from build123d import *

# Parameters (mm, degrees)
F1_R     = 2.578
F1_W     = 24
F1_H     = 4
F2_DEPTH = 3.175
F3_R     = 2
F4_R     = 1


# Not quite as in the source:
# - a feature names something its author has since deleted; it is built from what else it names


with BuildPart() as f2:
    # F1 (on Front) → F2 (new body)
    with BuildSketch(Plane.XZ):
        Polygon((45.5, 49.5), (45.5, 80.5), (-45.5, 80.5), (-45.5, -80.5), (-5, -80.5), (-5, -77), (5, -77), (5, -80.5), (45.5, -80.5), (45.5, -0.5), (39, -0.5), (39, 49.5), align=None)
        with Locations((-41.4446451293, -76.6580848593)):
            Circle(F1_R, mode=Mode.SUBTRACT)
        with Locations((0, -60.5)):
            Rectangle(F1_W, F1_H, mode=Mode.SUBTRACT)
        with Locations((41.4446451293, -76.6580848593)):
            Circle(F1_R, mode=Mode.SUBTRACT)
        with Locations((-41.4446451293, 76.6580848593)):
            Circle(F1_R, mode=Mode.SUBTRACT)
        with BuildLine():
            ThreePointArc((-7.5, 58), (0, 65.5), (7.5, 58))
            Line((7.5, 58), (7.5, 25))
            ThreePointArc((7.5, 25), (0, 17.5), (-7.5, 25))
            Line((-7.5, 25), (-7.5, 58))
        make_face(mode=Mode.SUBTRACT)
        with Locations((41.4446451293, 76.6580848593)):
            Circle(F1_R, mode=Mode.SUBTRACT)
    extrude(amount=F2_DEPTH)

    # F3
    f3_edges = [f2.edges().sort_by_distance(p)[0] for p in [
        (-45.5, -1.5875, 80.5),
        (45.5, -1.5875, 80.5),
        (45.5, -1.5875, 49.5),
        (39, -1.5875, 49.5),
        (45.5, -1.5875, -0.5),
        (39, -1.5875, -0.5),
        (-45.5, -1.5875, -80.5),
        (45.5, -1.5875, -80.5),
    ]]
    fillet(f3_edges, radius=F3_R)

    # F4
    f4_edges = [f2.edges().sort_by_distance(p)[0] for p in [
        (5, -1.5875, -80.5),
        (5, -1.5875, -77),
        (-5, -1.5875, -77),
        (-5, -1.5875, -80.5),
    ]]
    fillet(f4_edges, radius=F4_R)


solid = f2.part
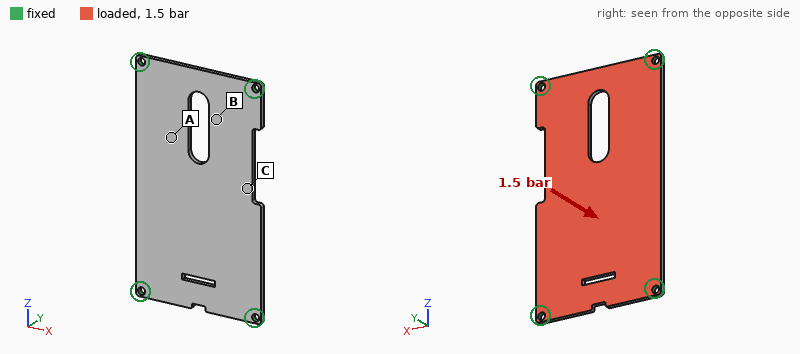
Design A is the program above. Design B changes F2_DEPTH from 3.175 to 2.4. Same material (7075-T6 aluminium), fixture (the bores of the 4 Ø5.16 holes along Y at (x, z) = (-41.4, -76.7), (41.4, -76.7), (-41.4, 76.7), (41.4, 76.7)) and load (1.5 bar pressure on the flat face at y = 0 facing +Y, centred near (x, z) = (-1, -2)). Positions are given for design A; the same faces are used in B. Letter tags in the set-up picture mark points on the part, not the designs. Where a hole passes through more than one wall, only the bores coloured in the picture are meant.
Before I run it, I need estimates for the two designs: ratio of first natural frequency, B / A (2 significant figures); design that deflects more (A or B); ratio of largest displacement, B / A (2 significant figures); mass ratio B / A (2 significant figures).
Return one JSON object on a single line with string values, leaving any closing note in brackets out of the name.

{"ratio of first natural frequency, B / A": "0.77", "design that deflects more": "B", "ratio of largest displacement, B / A": "2.3", "mass ratio B / A": "0.76"}
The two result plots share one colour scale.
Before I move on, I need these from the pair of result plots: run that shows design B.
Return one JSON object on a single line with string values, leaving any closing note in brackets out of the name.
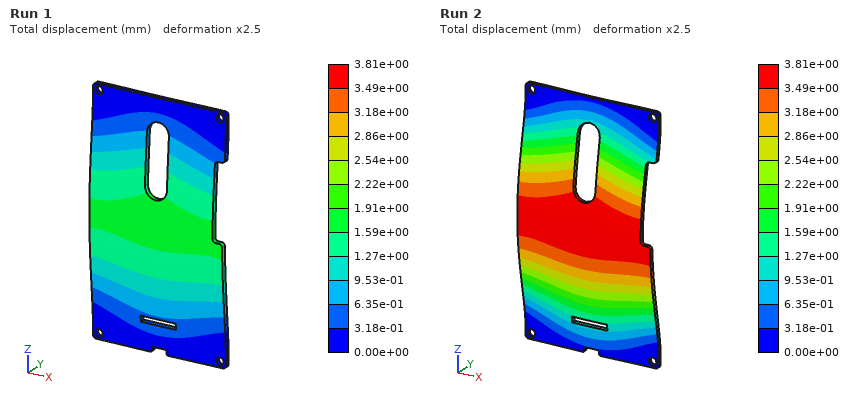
{"run that shows design B": "Run 2"}
